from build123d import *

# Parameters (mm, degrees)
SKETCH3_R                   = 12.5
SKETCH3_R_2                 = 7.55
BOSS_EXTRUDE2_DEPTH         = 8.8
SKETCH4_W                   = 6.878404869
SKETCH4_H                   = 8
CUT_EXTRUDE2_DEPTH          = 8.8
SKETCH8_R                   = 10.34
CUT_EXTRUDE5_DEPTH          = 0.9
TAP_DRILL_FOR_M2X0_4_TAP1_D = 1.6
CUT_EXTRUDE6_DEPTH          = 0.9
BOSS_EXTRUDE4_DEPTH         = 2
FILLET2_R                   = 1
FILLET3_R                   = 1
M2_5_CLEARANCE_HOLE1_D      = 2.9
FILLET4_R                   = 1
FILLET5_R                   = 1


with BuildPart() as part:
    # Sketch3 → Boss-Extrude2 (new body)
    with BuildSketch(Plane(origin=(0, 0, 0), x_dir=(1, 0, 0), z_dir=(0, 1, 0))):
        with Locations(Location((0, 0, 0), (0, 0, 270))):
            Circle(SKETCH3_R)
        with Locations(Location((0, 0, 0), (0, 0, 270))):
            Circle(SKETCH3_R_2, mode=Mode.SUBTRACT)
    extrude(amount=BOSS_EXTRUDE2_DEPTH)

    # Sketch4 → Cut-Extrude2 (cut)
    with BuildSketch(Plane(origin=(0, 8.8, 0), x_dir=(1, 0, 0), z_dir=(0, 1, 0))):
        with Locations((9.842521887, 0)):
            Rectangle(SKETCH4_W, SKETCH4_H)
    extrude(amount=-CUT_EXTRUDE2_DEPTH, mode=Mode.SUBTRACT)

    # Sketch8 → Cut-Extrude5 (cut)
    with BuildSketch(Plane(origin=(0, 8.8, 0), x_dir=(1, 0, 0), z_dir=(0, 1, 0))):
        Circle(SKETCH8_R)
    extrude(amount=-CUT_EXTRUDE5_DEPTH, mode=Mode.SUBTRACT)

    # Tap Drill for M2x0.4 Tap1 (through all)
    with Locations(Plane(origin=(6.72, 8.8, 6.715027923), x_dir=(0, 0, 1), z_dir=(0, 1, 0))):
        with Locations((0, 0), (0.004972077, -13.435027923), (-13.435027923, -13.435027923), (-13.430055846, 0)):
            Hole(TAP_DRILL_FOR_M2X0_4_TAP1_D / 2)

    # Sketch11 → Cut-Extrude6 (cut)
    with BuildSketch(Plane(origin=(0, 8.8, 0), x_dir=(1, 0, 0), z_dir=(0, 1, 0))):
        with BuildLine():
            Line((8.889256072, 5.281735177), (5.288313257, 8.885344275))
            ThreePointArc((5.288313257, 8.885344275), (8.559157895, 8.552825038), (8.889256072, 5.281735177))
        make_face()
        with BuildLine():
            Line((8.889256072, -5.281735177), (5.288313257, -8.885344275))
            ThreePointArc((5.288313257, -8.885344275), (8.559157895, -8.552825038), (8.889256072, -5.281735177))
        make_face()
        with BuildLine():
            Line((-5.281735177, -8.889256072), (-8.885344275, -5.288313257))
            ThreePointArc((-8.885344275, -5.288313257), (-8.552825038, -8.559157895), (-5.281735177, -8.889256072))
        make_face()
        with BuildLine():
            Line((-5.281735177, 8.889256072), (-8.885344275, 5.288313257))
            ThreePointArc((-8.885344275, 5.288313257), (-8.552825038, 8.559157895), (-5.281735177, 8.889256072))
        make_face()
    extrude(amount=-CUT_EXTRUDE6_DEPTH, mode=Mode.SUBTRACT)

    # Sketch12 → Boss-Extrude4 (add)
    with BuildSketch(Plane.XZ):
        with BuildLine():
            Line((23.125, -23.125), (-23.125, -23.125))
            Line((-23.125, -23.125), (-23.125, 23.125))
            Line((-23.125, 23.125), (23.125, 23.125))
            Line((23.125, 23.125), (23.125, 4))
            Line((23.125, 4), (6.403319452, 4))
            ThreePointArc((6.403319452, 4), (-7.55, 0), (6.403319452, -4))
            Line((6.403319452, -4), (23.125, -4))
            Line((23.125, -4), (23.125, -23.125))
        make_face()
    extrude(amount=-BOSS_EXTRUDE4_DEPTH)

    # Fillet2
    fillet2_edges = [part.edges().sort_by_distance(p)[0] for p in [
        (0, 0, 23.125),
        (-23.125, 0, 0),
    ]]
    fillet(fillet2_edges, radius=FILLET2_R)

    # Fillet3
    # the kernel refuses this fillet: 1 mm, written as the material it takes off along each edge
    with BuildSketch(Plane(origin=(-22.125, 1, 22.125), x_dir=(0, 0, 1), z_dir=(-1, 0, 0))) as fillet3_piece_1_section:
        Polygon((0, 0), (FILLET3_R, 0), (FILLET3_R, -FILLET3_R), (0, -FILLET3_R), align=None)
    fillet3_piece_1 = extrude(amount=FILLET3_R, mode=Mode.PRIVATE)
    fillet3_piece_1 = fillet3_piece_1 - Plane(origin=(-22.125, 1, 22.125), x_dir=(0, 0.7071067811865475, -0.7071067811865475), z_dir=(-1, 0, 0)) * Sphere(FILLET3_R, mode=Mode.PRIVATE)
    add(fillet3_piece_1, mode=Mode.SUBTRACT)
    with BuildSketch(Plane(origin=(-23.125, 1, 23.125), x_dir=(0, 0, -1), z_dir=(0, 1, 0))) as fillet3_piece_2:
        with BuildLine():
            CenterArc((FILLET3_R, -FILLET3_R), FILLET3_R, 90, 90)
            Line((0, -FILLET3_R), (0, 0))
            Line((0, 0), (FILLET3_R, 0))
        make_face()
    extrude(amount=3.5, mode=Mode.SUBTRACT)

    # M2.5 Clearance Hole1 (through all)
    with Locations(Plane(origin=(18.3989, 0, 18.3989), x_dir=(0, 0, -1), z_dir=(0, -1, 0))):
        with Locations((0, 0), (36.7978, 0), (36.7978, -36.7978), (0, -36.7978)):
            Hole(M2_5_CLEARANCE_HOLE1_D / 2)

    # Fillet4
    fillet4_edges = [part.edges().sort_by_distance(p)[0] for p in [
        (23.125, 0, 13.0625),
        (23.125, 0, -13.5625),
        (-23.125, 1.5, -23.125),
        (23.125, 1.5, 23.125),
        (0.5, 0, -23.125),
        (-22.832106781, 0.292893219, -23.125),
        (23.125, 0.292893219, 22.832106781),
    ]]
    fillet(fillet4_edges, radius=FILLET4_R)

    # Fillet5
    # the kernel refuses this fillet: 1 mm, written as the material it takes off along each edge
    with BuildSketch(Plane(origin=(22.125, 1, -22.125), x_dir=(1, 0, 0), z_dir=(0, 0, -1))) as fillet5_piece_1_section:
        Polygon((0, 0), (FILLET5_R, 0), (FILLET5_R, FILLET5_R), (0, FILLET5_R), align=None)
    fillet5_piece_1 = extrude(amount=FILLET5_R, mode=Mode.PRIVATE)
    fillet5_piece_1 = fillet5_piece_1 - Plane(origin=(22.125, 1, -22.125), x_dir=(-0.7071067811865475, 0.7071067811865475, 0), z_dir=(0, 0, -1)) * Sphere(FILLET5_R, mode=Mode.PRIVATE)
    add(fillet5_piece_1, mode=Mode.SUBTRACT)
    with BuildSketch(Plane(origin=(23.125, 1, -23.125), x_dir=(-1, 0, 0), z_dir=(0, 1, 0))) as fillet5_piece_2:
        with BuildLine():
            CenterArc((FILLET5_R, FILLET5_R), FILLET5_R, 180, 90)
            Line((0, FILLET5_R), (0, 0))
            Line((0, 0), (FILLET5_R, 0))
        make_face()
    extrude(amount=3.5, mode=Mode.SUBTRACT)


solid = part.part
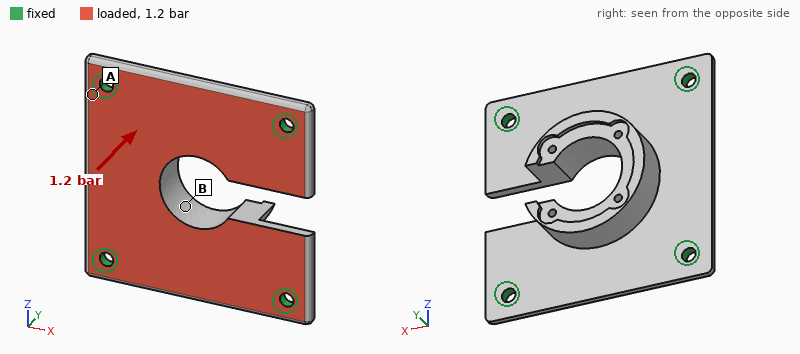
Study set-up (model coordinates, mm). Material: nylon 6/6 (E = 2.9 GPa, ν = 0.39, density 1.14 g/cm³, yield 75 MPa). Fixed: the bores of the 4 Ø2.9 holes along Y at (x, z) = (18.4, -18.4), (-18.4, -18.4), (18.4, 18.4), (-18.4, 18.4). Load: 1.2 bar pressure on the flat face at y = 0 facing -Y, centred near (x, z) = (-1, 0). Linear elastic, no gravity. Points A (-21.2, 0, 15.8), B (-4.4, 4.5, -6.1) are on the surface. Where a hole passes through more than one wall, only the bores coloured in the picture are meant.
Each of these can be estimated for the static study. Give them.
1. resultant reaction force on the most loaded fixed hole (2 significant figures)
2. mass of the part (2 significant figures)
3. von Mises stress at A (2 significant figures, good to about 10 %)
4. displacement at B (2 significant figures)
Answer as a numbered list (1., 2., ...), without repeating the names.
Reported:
1. 53 N
2. 6.0 g
3. 11 MPa
4. 0.26 mm
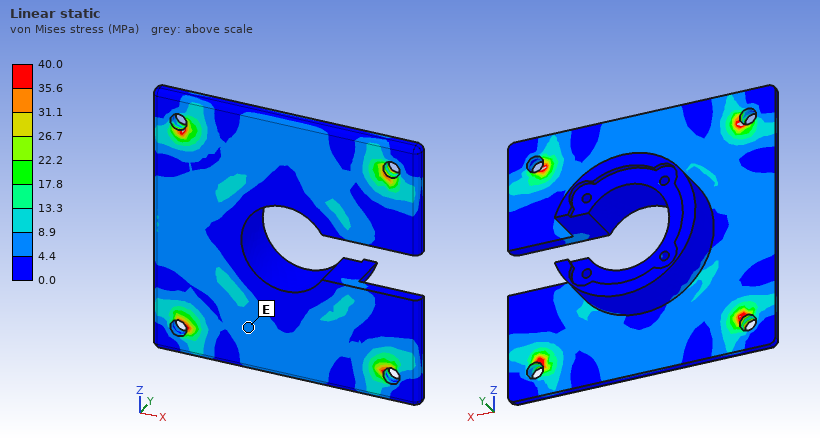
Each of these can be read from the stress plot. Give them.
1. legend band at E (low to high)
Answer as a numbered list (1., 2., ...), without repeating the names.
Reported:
1. 4.4 to 8.9 MPa
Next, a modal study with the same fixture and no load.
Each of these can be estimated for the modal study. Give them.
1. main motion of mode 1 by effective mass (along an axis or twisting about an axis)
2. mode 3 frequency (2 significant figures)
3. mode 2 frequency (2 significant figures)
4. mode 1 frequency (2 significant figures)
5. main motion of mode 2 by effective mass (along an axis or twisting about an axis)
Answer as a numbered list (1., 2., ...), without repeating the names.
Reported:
1. along Y
2. 2700 Hz
3. 2400 Hz
4. 1700 Hz
5. twisting about X
